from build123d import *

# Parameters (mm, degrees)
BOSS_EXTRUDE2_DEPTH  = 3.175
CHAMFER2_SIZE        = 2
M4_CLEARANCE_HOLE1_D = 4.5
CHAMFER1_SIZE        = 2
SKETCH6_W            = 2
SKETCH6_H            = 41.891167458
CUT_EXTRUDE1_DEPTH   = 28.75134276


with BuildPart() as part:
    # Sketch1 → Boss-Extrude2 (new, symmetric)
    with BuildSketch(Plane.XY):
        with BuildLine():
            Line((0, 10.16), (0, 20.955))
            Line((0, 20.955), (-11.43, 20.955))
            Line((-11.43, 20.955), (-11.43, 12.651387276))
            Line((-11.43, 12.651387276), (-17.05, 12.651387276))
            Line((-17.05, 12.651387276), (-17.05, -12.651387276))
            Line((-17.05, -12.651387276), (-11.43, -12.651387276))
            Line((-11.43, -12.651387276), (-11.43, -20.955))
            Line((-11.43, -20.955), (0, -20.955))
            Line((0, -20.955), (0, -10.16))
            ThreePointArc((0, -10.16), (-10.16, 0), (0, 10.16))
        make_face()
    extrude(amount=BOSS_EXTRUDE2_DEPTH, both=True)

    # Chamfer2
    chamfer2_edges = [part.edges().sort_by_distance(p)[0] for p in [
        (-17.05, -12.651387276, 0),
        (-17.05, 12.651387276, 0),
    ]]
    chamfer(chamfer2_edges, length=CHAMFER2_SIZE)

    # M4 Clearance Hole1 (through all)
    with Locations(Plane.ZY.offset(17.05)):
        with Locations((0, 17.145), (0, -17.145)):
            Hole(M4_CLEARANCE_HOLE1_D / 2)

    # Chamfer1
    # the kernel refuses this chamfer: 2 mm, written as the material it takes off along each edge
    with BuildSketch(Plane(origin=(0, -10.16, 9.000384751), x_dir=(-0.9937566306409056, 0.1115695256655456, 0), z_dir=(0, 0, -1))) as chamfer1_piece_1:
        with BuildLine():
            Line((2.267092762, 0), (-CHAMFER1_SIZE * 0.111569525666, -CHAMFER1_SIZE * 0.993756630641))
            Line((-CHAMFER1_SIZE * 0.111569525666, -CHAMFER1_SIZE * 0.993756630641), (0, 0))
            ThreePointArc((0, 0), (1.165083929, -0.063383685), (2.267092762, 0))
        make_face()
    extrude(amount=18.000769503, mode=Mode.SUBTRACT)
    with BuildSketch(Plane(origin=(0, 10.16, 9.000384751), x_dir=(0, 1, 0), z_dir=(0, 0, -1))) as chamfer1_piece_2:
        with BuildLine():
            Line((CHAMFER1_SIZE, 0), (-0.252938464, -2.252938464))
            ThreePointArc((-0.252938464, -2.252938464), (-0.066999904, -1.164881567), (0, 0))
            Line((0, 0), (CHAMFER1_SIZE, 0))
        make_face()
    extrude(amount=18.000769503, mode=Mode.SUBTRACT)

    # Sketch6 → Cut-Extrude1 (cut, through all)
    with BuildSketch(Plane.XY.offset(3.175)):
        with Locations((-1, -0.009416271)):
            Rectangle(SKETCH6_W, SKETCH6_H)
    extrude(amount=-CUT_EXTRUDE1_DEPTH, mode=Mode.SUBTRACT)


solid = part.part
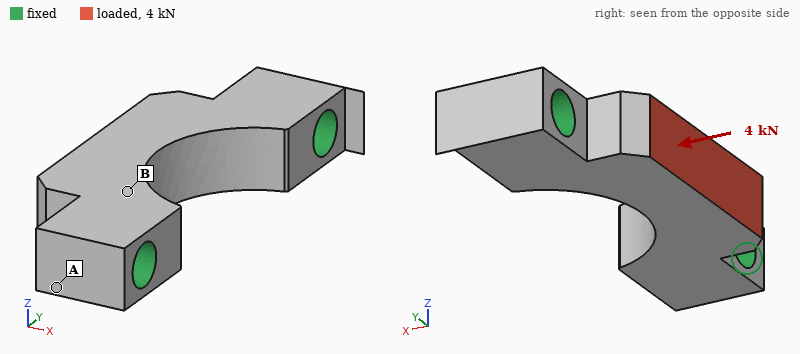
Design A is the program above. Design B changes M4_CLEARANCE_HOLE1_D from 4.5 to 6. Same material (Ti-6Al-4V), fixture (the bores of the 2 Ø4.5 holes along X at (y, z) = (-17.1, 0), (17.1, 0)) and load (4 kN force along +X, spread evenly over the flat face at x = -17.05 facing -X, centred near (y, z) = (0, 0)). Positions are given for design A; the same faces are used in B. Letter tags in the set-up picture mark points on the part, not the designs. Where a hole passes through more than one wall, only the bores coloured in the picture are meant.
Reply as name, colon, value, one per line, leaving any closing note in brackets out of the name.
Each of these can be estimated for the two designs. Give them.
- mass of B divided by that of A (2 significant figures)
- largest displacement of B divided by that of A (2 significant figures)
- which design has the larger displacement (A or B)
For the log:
mass of B divided by that of A: 0.90
largest displacement of B divided by that of A: 0.91
which design has the larger displacement: A
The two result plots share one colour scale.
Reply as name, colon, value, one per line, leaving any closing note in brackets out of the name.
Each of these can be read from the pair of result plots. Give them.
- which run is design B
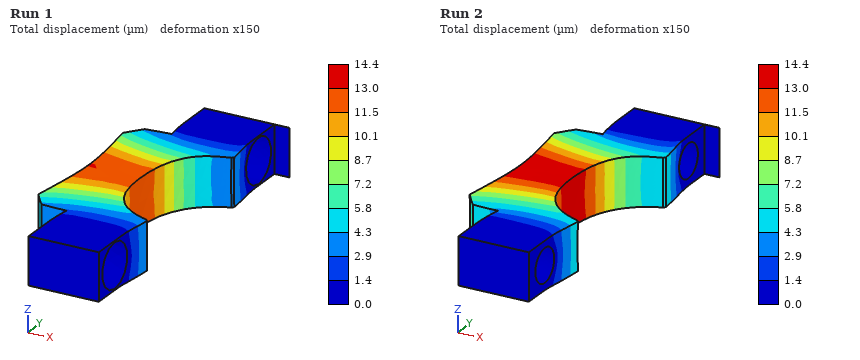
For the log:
which run is design B: Run 1
